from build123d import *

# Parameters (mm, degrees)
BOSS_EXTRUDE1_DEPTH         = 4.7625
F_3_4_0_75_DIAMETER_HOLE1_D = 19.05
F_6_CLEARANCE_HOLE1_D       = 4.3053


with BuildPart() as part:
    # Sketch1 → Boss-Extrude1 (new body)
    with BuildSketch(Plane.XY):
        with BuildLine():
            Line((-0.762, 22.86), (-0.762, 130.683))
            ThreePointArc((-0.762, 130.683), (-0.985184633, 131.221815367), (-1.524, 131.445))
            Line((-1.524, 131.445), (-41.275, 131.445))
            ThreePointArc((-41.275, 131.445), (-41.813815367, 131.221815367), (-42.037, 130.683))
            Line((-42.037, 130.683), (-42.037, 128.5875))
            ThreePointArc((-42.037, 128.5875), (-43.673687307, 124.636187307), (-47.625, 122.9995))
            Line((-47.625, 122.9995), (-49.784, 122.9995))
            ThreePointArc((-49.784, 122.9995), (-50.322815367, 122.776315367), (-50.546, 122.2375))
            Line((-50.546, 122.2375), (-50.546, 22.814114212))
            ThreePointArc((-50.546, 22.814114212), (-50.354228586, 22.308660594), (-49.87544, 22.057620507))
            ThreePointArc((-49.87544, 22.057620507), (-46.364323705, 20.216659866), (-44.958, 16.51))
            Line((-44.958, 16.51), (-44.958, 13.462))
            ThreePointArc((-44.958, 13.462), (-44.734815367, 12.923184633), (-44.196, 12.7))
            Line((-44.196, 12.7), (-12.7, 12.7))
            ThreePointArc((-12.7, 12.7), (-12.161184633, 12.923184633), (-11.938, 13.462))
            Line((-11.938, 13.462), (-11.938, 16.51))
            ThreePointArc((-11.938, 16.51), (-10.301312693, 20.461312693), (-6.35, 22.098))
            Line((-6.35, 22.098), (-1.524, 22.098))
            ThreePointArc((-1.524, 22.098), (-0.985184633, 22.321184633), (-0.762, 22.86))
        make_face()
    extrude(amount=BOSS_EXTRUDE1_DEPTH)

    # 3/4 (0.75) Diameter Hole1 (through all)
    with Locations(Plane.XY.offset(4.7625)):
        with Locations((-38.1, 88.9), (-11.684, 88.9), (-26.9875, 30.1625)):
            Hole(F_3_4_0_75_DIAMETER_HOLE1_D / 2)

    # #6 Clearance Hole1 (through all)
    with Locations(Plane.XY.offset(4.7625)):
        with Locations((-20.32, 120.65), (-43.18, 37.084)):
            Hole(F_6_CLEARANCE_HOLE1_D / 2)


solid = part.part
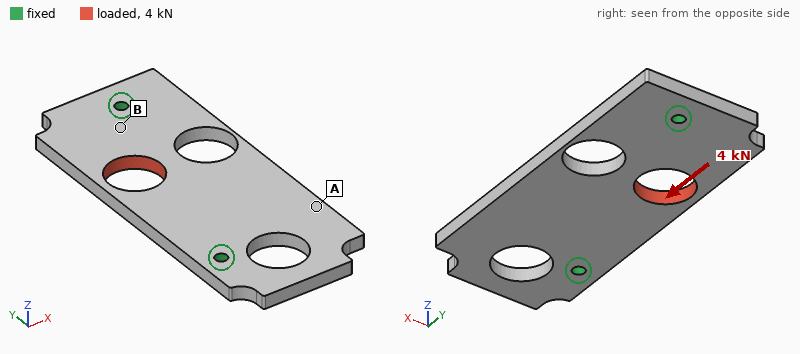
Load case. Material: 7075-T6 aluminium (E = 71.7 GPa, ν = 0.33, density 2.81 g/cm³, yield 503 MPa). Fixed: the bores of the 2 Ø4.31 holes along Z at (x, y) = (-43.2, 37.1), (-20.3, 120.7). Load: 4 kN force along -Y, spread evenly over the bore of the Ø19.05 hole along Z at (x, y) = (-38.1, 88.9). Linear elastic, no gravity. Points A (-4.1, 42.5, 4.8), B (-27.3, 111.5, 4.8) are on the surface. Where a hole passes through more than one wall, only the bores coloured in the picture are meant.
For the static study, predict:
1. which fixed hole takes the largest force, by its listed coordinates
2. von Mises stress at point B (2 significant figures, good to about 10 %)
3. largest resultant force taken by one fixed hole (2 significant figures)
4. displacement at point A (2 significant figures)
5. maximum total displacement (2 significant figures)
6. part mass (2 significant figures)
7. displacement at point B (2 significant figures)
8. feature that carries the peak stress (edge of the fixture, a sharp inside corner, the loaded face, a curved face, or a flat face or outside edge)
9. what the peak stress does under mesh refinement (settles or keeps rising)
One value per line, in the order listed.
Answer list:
(-20.3, 120.7)
22 MPa
2.3 kN
16 µm
28 µm
64 g
9.7 µm
edge of the fixture
keeps rising
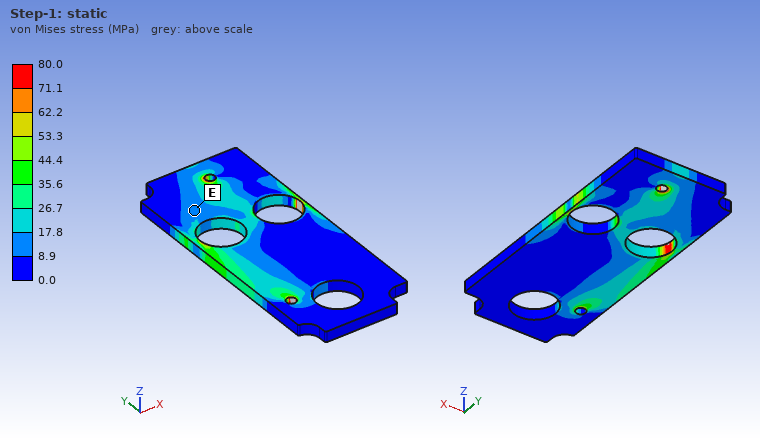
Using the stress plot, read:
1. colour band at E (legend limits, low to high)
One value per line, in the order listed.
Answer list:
8.9 to 17.8 MPa
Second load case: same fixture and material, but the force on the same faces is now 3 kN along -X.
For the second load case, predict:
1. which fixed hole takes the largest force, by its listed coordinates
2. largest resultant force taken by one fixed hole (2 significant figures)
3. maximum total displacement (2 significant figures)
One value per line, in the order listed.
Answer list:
(-20.3, 120.7)
1.8 kN
40 µm
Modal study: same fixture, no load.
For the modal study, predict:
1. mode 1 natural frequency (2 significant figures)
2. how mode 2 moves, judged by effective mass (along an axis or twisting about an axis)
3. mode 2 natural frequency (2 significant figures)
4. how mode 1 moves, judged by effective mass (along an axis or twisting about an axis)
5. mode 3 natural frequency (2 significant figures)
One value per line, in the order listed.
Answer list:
1700 Hz
along Z
2700 Hz
along Z
3600 Hz
